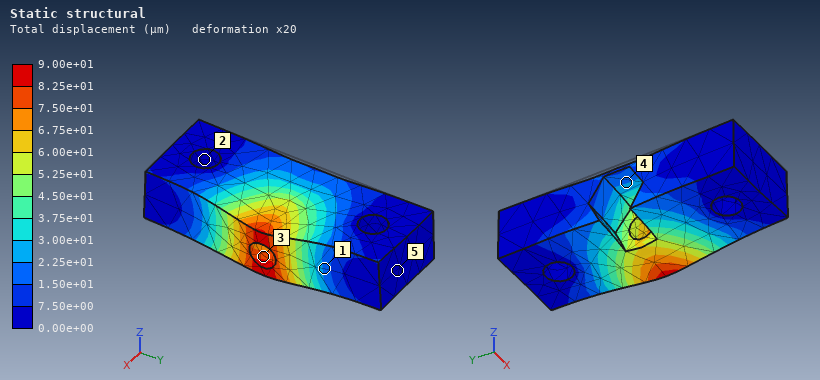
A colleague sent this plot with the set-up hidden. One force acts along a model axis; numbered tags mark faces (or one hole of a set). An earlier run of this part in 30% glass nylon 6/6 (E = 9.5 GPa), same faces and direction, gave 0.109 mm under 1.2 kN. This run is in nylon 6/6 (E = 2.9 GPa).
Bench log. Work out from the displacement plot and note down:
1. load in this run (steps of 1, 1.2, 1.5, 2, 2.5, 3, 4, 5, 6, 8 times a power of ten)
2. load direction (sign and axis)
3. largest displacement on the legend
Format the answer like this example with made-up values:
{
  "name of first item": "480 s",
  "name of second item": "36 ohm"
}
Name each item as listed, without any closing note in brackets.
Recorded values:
{
  "load in this run": "300 N",
  "load direction": "-Z",
  "largest displacement on the legend": "9.00e+01 µm"
}
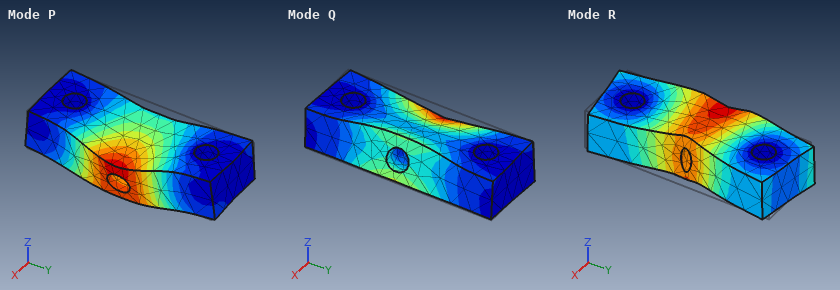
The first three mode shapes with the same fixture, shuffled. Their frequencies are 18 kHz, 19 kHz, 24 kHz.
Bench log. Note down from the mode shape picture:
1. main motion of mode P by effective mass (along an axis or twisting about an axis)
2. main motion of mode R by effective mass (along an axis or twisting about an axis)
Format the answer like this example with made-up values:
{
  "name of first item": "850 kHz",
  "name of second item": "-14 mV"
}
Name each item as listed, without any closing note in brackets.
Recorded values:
{
  "main motion of mode P by effective mass": "along Z",
  "main motion of mode R by effective mass": "along X"
}
